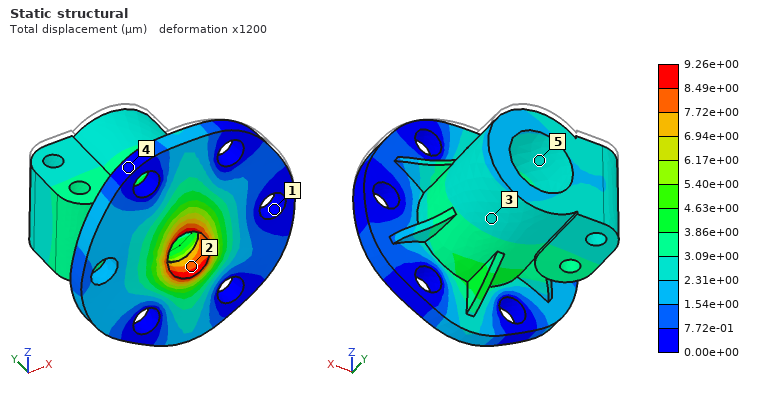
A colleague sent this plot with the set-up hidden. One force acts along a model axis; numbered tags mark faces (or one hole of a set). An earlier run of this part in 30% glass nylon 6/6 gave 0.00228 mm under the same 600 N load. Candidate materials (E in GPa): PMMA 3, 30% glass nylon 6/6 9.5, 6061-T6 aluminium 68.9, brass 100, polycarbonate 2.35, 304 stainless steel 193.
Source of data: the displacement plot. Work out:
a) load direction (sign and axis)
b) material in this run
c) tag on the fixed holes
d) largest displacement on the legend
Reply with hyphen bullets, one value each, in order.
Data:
- -Z
- polycarbonate
- 1
- 9.26e+00 µm
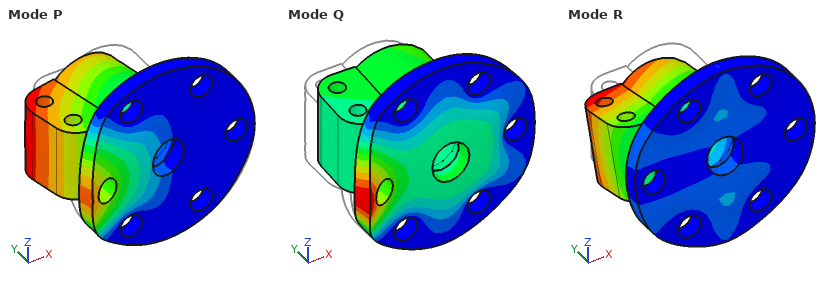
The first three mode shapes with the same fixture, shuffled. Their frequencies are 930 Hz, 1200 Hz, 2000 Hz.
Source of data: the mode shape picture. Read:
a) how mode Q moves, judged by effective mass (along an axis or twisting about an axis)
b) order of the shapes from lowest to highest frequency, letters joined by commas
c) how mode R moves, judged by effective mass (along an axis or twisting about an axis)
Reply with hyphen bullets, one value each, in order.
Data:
- along Y
- P, R, Q
- along Z
